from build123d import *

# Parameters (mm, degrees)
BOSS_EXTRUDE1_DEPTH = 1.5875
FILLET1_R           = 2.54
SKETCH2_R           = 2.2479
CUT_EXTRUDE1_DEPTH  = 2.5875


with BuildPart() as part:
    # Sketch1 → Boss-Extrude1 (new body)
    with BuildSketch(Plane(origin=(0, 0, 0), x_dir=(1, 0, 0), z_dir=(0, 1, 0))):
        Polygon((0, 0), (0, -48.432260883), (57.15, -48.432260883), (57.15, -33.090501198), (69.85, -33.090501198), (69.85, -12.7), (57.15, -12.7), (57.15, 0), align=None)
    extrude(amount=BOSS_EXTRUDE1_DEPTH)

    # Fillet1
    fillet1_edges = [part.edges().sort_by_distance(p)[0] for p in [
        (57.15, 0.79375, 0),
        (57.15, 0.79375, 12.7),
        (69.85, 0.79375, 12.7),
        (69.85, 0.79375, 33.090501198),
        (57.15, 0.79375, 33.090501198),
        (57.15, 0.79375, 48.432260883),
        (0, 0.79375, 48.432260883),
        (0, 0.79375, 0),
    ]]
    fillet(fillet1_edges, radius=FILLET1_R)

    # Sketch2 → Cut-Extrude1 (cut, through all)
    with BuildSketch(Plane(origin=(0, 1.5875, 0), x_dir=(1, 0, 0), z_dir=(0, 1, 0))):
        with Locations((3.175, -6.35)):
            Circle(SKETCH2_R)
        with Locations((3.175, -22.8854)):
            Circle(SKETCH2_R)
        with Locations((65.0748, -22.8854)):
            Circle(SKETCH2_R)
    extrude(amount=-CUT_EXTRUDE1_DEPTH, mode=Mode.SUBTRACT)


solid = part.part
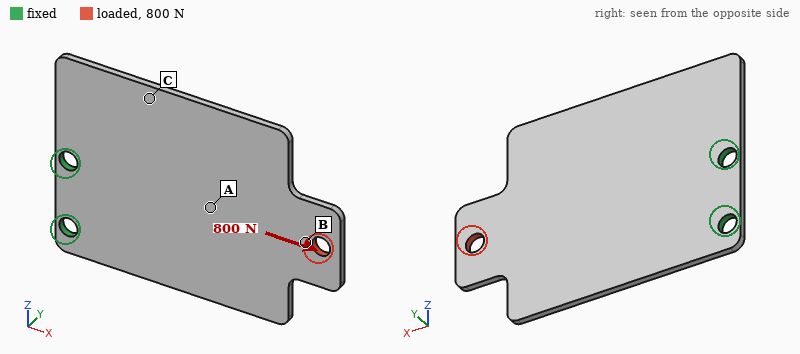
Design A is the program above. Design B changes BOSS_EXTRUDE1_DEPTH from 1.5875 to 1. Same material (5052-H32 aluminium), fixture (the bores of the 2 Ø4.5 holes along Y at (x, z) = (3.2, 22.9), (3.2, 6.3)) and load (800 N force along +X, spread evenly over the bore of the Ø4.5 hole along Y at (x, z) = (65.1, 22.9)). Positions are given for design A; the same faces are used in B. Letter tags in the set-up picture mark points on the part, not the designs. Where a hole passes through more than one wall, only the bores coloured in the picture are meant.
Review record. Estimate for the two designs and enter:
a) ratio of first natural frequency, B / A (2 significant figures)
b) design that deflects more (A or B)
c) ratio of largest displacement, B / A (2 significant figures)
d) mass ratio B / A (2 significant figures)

0.64
B
1.6
0.63
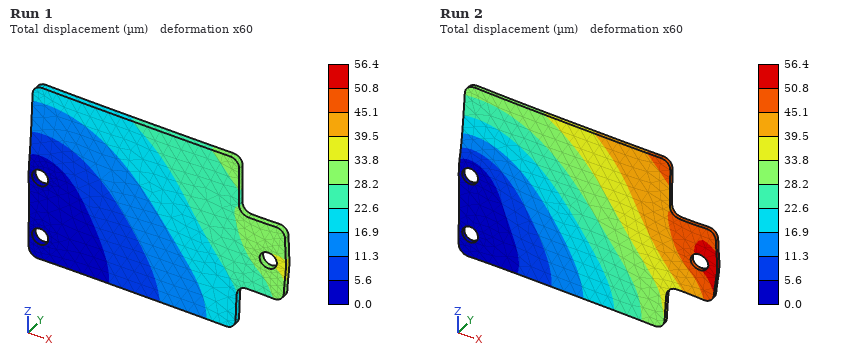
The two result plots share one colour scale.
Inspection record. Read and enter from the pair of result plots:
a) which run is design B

Run 2
